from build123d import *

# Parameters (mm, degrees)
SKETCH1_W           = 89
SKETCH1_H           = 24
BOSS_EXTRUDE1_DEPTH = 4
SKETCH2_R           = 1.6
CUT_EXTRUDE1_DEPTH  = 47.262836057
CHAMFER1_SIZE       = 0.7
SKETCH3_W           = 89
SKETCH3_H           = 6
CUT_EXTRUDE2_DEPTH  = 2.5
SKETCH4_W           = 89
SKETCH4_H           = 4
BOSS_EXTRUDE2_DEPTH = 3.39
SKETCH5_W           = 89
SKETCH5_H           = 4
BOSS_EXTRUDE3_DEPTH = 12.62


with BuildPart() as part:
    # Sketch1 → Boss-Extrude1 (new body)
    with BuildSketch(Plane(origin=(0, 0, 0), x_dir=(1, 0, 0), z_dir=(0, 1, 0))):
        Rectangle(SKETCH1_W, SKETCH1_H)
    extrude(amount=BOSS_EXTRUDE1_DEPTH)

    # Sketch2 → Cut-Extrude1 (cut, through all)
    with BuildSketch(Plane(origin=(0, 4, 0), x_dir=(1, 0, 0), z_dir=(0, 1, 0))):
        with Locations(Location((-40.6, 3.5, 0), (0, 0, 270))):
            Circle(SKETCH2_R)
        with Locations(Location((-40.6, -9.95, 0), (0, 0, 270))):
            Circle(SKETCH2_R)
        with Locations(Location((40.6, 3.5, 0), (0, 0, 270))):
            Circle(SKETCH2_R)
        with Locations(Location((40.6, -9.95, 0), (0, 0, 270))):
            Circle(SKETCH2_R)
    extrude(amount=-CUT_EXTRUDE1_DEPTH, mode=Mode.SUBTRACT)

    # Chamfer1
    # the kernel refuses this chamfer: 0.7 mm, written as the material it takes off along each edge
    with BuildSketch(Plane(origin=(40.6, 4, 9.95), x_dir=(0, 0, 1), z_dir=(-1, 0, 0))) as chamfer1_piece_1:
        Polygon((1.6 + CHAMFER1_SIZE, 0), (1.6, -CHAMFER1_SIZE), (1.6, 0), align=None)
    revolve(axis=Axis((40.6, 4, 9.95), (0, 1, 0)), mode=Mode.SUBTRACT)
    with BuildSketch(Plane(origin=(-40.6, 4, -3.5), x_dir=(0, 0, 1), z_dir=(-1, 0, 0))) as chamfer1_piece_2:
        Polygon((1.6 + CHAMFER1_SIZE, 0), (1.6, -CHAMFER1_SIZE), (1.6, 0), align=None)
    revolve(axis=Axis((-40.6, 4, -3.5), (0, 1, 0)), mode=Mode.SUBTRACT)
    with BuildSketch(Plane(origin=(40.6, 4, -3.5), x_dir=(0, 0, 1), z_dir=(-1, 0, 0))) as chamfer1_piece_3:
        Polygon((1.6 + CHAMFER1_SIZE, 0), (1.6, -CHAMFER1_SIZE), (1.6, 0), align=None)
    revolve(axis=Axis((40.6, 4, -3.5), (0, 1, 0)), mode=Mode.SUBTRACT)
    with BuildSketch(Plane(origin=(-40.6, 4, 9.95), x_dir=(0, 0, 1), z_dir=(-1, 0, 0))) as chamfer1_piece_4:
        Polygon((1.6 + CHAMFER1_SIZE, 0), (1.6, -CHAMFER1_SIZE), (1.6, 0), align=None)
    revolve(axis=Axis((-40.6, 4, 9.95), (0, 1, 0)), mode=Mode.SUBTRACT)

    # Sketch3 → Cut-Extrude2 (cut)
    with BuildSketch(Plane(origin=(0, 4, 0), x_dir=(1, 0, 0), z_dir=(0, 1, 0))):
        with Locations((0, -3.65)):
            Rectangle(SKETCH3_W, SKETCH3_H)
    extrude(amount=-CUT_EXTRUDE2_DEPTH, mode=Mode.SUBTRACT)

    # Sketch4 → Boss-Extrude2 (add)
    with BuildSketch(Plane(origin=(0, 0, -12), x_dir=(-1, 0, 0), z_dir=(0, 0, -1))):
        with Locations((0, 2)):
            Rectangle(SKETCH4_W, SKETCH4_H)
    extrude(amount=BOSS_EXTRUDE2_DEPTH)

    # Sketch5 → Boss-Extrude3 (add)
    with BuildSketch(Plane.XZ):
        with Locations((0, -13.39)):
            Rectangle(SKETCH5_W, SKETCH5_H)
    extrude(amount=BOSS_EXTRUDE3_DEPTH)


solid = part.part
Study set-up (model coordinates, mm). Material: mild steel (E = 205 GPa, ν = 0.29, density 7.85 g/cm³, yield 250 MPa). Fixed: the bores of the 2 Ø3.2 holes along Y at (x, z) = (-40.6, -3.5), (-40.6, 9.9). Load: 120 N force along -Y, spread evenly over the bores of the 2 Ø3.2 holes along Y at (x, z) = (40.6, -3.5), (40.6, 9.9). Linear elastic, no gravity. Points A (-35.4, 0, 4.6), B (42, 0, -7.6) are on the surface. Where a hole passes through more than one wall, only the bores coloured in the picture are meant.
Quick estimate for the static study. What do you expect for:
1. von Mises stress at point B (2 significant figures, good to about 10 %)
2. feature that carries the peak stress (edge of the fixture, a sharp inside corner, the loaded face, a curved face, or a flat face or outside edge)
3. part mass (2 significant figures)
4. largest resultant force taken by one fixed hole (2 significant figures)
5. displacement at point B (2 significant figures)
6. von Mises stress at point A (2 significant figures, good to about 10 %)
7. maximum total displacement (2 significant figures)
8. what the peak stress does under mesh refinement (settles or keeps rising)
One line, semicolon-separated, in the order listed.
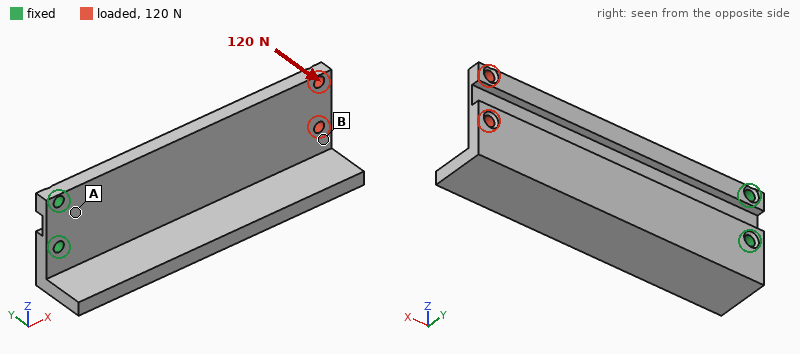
22 MPa; edge of the fixture; 100 g; 170 N; 0.31 mm; 77 MPa; 0.36 mm; keeps rising
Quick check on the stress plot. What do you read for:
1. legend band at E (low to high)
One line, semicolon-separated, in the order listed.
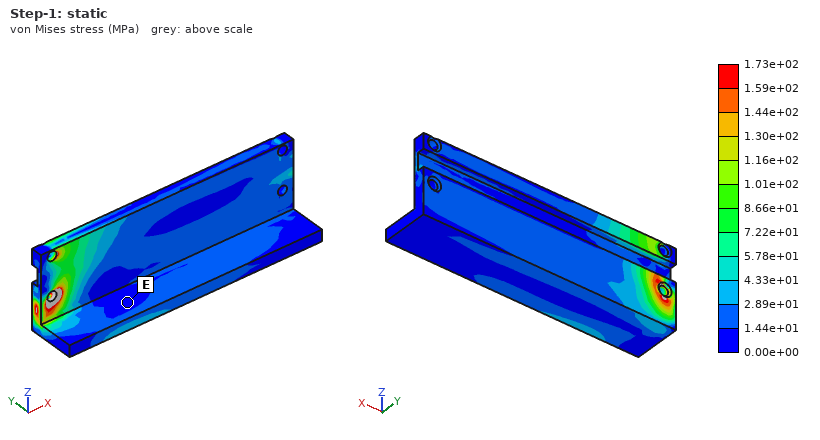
0.00e+00 to 1.44e+01 MPa
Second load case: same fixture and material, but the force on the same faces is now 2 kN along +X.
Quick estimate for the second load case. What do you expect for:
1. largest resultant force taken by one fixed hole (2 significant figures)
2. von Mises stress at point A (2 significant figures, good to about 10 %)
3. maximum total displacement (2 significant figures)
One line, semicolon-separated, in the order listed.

1.0 kN; 24 MPa; 42 µm
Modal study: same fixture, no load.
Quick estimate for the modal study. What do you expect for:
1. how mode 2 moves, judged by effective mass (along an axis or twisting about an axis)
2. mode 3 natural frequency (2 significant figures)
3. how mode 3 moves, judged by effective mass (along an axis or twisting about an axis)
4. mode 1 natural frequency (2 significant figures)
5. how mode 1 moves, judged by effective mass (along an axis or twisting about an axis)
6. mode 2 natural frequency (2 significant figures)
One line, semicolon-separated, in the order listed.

along Z; 2100 Hz; along Z; 540 Hz; along Y; 1800 Hz
